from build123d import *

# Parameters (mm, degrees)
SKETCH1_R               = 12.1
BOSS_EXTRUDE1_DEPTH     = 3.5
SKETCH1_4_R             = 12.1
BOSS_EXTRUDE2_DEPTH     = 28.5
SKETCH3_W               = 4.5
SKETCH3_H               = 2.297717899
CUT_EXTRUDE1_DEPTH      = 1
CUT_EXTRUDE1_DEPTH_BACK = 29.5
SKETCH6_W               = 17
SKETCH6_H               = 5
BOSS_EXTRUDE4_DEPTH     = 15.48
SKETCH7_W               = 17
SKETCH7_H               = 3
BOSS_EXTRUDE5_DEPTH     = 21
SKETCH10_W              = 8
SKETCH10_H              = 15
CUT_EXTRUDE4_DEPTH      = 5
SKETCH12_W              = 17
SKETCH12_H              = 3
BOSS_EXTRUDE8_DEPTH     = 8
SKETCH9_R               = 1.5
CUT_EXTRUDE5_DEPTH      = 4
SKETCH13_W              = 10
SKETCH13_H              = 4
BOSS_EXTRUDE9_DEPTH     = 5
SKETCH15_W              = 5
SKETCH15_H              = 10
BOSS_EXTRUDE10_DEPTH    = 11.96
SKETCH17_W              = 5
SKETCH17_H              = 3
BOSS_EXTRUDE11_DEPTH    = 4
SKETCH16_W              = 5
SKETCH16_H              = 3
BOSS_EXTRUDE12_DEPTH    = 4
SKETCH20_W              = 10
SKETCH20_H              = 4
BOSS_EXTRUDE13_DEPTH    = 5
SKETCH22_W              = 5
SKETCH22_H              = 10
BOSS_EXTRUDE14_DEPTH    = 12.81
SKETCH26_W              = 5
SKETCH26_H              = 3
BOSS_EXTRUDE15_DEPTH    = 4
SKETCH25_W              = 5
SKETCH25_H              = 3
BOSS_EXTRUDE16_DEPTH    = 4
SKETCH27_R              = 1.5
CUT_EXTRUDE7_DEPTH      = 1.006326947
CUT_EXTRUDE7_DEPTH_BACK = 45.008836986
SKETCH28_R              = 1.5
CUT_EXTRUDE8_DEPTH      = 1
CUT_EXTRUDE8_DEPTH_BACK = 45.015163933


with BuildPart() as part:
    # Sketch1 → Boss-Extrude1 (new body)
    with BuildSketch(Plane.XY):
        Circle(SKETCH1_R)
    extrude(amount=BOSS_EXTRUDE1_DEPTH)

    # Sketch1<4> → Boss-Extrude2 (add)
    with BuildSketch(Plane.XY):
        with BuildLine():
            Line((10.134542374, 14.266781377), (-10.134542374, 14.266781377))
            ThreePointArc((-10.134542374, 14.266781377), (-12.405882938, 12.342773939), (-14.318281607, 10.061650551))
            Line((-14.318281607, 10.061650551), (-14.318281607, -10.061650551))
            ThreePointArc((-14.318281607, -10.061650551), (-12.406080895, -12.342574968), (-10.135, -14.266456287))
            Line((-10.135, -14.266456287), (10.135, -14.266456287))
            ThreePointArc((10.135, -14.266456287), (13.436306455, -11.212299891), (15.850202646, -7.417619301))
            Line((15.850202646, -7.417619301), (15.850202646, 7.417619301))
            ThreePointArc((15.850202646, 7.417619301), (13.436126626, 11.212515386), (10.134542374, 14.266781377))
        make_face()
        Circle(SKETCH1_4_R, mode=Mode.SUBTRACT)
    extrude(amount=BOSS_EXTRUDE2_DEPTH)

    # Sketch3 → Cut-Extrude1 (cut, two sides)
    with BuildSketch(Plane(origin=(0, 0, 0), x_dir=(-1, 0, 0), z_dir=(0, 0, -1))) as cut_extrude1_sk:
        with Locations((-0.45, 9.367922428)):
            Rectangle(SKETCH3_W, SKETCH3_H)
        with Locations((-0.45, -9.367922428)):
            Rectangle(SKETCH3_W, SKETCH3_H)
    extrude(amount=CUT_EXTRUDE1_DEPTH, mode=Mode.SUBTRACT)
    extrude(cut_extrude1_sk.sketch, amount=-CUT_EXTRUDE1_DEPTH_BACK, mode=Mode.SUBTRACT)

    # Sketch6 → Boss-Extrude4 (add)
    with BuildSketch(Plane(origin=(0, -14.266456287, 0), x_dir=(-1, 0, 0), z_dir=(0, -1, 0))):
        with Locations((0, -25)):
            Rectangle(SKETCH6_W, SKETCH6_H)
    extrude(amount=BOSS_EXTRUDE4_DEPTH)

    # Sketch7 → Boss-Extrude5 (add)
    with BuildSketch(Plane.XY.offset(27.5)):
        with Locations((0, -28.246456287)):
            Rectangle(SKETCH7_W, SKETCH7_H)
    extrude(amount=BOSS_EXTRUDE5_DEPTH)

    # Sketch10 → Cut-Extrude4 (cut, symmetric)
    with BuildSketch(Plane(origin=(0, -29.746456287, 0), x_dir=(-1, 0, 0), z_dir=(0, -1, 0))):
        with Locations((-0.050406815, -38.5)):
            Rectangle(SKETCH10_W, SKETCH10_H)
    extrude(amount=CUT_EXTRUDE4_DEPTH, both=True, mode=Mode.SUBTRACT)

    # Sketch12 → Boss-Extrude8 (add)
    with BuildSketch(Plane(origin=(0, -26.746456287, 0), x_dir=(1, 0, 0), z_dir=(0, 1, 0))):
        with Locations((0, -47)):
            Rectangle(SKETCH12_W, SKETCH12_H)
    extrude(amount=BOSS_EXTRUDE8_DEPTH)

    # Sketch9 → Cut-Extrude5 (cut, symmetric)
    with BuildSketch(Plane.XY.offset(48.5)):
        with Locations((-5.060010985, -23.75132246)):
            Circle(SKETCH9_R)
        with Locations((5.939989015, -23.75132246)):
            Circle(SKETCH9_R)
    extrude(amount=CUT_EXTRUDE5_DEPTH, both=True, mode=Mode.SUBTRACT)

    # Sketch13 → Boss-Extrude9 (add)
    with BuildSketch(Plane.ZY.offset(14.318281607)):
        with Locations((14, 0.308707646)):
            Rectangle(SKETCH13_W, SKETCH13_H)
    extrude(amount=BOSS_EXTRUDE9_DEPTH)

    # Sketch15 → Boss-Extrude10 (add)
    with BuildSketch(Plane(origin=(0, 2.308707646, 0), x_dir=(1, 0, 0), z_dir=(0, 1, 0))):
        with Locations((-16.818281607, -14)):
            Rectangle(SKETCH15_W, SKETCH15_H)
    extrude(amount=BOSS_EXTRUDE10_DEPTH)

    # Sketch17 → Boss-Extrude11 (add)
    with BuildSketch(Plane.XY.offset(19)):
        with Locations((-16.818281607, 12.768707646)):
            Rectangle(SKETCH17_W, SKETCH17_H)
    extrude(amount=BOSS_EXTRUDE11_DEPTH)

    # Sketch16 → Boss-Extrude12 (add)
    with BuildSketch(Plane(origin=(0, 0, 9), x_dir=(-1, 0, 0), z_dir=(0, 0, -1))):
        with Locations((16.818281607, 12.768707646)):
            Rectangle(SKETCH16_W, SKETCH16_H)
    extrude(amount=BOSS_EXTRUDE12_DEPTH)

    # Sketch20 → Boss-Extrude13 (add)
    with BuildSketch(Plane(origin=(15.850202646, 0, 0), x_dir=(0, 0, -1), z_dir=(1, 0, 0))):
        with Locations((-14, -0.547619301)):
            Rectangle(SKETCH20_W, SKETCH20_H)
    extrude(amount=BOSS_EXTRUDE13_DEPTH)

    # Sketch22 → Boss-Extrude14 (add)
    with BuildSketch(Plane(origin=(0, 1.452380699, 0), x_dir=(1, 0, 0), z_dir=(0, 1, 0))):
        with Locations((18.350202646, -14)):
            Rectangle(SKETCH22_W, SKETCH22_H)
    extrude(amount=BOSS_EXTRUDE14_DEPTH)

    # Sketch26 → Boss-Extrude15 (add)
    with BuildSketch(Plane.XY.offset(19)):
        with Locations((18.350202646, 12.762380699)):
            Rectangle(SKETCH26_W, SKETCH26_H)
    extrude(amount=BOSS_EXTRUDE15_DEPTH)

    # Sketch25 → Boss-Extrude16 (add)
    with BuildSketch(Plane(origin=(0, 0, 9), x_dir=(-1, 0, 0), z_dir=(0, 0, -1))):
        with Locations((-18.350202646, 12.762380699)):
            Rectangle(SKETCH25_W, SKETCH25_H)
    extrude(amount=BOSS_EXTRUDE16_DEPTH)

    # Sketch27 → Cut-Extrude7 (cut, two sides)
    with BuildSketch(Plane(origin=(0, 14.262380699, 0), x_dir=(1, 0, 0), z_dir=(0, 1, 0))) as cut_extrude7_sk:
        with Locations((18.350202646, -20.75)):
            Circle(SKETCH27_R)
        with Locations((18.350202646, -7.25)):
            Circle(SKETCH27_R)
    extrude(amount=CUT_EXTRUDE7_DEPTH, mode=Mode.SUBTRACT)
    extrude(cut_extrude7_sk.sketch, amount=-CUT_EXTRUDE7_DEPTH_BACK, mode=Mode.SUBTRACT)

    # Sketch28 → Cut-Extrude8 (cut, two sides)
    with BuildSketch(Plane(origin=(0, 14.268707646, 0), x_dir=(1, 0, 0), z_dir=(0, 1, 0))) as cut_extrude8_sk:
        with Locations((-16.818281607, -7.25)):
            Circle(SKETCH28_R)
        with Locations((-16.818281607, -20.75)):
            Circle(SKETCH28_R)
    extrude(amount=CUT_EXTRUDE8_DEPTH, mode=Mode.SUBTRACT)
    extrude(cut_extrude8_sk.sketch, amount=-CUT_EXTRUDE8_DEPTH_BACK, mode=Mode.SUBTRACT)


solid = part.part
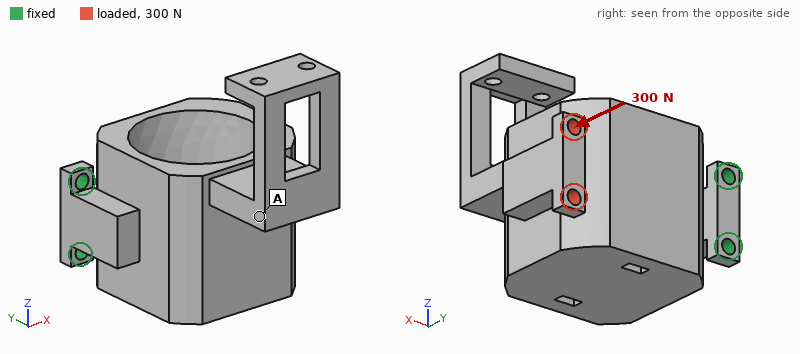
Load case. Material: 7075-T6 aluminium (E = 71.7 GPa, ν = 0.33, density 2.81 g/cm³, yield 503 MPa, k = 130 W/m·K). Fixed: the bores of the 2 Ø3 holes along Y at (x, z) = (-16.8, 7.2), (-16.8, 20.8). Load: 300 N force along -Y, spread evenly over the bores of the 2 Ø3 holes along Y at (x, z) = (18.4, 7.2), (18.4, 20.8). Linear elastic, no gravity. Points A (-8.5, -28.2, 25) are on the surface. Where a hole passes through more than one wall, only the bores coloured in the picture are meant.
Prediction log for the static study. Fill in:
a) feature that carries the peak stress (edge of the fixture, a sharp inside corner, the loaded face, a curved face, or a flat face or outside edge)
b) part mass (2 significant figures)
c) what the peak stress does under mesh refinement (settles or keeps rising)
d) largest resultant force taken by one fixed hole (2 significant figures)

edge of the fixture
44 g
keeps rising
170 N
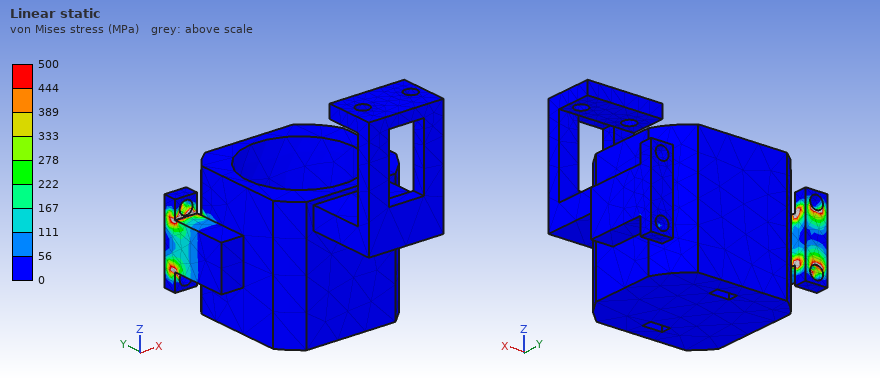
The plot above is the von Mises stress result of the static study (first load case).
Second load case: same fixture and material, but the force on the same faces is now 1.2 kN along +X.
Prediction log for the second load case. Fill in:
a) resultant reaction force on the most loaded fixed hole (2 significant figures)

600 N
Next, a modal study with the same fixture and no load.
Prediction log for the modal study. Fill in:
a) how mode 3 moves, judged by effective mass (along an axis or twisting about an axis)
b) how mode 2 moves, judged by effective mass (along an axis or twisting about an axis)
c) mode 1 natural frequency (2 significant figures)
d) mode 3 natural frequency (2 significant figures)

twisting about X
along Z
660 Hz
2000 Hz
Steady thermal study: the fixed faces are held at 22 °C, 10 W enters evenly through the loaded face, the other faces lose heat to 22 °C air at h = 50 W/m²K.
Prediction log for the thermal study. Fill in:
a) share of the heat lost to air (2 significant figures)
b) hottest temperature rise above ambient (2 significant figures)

49 %
41 K
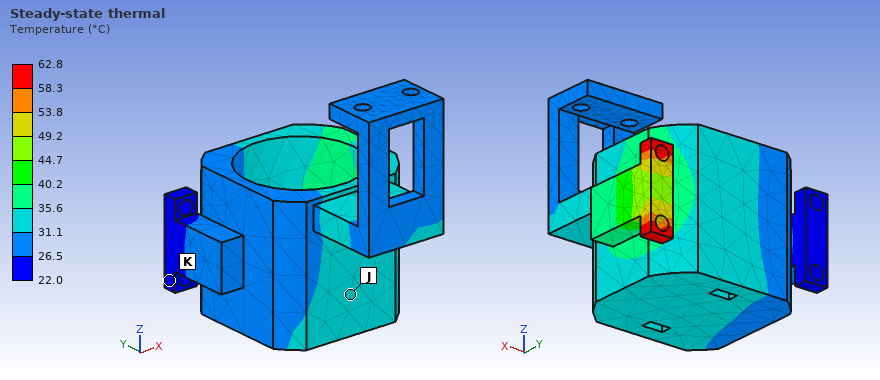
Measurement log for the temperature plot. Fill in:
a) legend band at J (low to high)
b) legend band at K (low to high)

31.1 to 35.6 °C
22.0 to 26.5 °C
